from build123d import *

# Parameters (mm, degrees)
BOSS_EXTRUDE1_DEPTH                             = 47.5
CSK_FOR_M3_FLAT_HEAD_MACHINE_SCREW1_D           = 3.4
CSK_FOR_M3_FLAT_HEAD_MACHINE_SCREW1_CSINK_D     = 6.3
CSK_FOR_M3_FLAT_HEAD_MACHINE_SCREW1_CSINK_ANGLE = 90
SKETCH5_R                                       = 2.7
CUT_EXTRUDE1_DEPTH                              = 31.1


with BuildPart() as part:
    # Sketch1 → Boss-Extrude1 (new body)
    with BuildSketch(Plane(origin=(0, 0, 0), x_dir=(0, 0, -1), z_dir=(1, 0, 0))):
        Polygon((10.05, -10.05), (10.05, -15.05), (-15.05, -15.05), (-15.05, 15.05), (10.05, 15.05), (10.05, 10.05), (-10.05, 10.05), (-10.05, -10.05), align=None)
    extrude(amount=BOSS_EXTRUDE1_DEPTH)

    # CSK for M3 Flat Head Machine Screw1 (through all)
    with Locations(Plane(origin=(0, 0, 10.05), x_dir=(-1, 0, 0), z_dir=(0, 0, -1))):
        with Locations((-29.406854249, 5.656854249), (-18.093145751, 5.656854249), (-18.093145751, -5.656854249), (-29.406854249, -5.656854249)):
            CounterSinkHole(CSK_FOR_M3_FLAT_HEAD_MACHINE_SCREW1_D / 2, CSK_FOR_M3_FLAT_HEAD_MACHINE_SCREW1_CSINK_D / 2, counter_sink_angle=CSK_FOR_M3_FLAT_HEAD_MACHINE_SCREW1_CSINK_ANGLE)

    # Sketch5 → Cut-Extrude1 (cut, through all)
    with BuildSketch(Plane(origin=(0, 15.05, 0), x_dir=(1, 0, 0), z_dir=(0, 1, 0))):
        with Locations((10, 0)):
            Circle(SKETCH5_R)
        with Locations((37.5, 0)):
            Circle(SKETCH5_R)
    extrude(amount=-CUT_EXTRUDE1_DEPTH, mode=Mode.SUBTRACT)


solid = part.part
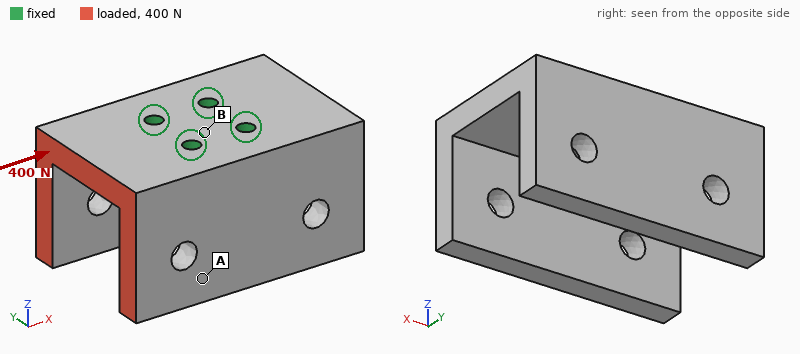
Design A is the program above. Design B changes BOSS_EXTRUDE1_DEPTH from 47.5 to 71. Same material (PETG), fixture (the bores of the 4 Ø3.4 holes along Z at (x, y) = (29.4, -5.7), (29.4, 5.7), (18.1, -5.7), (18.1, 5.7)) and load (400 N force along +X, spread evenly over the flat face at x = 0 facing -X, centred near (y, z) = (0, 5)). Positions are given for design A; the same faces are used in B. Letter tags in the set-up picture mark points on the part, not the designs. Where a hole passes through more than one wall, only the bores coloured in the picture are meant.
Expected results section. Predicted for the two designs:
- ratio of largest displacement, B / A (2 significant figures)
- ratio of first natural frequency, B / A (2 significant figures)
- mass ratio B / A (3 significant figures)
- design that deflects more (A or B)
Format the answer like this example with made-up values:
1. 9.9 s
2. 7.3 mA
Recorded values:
1. 1.4
2. 0.65
3. 1.52
4. B
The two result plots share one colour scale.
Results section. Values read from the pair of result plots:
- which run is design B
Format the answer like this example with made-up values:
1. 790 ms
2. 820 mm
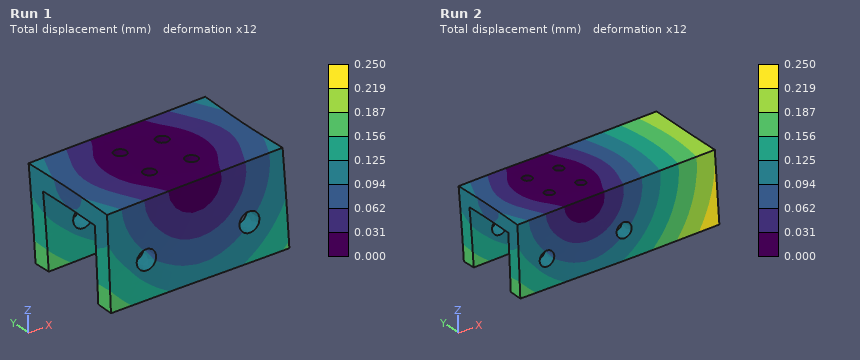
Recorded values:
1. Run 2
